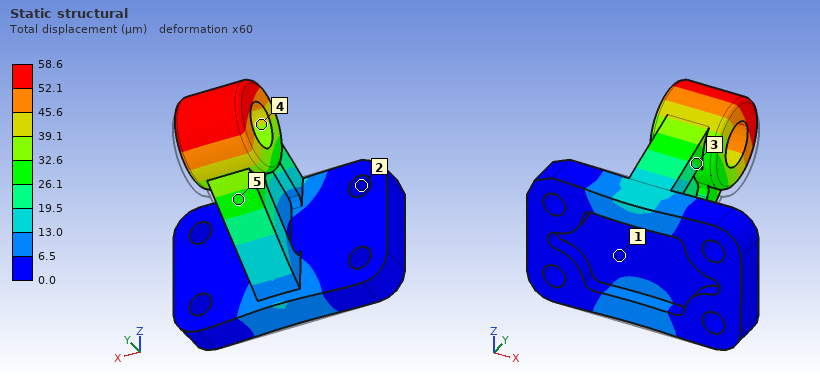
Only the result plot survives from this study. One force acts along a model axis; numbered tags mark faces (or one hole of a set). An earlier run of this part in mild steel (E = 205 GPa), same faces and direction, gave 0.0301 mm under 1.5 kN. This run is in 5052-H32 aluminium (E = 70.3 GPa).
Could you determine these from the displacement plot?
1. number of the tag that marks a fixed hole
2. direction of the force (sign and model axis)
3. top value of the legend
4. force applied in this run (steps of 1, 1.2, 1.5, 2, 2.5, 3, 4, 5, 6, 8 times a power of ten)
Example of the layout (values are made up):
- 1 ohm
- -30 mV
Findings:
- 2
- +Z
- 58.6 µm
- 1 kN
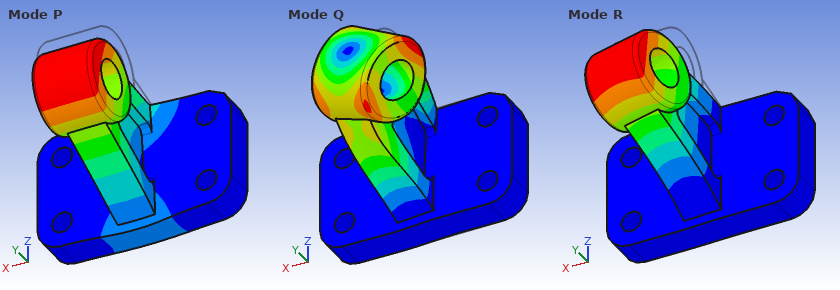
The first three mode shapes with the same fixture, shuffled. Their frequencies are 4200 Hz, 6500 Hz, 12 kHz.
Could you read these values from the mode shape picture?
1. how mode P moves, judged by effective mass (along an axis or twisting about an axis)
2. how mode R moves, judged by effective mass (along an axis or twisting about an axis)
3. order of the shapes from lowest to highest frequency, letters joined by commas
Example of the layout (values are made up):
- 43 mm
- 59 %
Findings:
- along Z
- along X
- R, P, Q
